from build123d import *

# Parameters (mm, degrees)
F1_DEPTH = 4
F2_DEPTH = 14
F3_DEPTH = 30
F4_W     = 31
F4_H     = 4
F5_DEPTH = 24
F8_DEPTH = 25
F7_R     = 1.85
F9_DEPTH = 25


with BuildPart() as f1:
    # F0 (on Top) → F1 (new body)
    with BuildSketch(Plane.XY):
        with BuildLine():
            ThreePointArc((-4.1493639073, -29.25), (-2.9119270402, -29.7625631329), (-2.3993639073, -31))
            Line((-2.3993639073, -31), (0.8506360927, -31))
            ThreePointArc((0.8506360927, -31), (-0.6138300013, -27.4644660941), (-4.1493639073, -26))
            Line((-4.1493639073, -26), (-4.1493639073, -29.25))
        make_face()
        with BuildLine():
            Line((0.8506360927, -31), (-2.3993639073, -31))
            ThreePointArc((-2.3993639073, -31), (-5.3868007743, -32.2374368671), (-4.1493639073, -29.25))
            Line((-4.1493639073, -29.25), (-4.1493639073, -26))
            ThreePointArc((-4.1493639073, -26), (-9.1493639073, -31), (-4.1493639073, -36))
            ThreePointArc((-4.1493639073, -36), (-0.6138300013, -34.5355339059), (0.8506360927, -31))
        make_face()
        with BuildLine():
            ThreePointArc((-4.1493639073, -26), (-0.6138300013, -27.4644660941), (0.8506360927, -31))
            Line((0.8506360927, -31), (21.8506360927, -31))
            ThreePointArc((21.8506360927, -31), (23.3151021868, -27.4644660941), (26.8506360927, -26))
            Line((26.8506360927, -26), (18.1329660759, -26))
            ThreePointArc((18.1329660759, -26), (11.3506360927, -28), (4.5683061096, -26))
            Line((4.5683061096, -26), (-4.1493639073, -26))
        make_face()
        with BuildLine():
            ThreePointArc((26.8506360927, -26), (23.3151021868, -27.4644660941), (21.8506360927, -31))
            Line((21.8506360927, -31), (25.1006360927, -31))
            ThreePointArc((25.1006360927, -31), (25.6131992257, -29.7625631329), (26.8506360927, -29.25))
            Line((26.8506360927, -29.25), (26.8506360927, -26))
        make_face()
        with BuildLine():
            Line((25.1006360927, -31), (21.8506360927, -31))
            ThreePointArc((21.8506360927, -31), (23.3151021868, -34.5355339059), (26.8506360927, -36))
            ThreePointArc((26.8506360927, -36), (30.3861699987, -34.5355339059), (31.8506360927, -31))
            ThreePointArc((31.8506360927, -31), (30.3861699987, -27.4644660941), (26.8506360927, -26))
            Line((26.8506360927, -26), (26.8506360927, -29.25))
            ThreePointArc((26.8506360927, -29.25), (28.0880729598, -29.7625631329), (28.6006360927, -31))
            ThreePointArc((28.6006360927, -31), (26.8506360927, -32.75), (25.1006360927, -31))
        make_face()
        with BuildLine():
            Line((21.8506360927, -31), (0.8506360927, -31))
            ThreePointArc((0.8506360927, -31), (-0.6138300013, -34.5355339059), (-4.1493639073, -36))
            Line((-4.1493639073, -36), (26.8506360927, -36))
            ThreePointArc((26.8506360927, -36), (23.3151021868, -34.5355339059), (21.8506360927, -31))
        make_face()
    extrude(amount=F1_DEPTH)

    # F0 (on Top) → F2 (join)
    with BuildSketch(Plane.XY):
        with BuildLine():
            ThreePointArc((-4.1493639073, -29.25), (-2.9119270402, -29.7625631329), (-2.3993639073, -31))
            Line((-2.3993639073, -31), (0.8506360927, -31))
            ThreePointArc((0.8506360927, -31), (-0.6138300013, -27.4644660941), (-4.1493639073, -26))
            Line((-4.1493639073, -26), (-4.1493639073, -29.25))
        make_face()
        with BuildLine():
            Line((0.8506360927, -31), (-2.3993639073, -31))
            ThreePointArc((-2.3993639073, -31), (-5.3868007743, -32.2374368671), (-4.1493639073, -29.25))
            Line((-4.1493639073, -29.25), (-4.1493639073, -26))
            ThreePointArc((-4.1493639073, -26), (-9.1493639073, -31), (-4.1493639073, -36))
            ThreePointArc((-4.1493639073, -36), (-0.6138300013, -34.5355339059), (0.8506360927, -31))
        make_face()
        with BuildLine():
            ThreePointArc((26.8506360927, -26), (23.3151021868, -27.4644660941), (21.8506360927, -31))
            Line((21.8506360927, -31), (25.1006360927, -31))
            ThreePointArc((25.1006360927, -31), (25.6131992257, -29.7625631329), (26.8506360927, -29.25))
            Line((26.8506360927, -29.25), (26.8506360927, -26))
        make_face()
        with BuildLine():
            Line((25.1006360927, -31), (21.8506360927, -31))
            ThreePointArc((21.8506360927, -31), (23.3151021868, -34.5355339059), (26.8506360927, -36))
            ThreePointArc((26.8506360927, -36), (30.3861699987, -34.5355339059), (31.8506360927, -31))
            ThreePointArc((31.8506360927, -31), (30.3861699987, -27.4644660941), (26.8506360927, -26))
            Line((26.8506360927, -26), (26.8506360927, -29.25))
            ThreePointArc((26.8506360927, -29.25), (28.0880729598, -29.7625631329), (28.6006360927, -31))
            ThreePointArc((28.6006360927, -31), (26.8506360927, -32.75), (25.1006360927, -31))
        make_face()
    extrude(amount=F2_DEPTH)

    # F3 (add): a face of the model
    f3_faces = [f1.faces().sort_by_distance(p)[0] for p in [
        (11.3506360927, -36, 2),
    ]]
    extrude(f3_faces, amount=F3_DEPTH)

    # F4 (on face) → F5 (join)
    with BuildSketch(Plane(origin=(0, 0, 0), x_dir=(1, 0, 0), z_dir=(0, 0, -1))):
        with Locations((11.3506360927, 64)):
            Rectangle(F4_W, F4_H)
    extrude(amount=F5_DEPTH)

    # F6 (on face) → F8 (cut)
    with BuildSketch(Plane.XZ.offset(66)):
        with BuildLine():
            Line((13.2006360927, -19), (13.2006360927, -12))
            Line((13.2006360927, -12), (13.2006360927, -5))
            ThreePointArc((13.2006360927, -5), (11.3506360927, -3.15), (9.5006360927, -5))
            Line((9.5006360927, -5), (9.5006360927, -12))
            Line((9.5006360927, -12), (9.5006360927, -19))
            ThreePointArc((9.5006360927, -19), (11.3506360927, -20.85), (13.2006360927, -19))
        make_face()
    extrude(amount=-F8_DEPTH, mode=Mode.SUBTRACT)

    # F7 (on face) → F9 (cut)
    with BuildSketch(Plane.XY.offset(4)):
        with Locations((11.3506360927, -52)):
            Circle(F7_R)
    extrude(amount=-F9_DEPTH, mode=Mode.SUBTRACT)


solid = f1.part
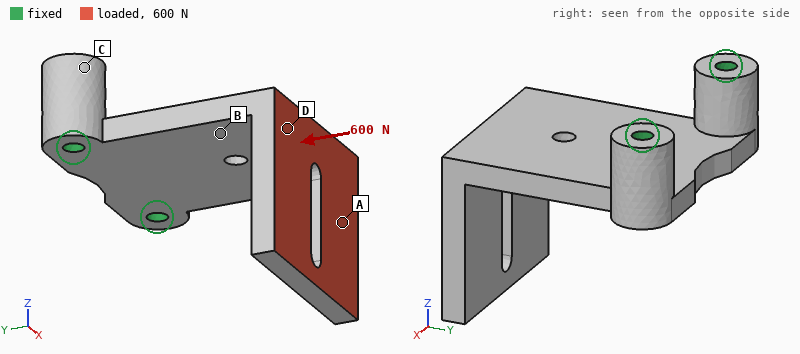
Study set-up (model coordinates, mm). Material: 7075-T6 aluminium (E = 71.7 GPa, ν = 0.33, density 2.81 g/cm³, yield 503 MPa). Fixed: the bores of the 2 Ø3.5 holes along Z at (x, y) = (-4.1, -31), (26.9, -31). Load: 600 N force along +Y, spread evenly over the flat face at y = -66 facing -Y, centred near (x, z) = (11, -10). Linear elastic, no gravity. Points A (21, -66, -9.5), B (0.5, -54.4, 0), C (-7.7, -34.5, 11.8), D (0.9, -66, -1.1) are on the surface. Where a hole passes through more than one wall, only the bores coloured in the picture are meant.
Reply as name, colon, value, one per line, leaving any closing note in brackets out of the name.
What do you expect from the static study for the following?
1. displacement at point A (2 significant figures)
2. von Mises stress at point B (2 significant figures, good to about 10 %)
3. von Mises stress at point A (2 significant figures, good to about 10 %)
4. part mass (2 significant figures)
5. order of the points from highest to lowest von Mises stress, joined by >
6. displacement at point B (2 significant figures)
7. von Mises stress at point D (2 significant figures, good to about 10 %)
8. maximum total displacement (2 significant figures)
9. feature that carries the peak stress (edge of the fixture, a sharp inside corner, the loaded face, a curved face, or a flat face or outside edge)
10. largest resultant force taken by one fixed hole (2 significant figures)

displacement at point A: 0.45 mm
von Mises stress at point B: 91 MPa
von Mises stress at point A: 31 MPa
part mass: 26 g
order of the points from highest to lowest von Mises stress, joined by >: B > D > A > C
displacement at point B: 0.17 mm
von Mises stress at point D: 59 MPa
maximum total displacement: 0.71 mm
feature that carries the peak stress: a curved face
largest resultant force taken by one fixed hole: 320 N
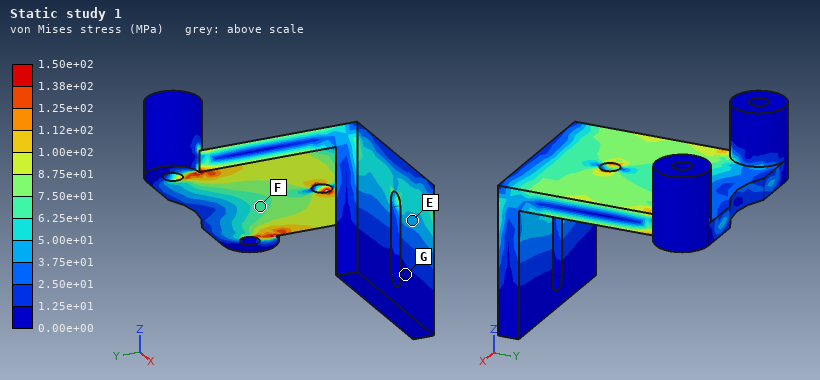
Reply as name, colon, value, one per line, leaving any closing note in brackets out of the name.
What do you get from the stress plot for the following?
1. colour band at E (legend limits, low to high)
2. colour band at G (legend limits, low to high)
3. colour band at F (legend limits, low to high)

colour band at E: 3.75e+01 to 5.00e+01 MPa
colour band at G: 0.00e+00 to 1.25e+01 MPa
colour band at F: 6.25e+01 to 7.50e+01 MPa
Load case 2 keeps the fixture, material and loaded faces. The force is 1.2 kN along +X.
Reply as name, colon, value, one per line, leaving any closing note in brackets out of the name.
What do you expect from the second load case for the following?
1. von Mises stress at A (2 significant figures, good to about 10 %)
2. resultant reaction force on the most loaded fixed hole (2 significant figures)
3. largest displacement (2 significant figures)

von Mises stress at A: 18 MPa
resultant reaction force on the most loaded fixed hole: 1.6 kN
largest displacement: 0.54 mm
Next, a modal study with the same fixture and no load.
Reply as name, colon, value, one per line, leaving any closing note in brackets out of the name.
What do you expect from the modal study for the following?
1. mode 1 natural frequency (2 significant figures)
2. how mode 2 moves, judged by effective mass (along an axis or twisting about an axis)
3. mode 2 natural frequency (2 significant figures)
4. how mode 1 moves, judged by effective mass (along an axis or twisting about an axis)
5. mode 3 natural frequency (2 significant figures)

mode 1 natural frequency: 1300 Hz
how mode 2 moves, judged by effective mass: along X
mode 2 natural frequency: 2600 Hz
how mode 1 moves, judged by effective mass: along Z
mode 3 natural frequency: 3900 Hz
